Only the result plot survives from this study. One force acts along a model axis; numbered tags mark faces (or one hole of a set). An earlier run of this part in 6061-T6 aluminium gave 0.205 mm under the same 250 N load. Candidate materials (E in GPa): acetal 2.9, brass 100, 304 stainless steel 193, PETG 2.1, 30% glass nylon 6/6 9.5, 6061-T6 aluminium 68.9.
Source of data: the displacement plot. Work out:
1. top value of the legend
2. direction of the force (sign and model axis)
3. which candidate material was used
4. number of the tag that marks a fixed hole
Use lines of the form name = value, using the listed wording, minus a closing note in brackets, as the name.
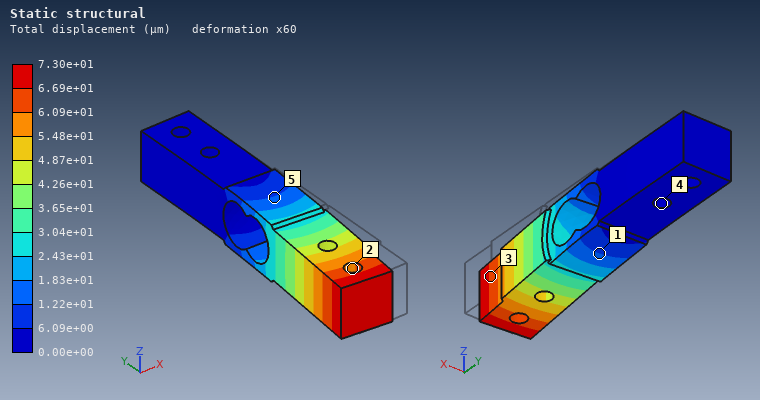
top value of the legend = 7.30e+01 µm
direction of the force = -X
which candidate material was used = 304 stainless steel
number of the tag that marks a fixed hole = 4
